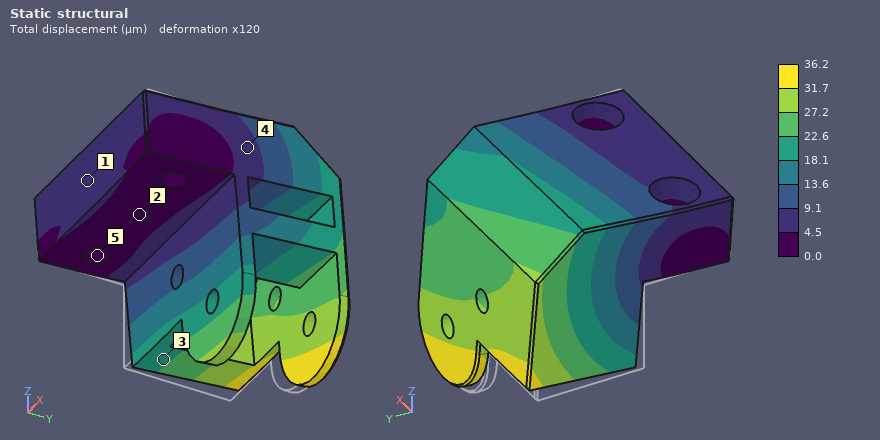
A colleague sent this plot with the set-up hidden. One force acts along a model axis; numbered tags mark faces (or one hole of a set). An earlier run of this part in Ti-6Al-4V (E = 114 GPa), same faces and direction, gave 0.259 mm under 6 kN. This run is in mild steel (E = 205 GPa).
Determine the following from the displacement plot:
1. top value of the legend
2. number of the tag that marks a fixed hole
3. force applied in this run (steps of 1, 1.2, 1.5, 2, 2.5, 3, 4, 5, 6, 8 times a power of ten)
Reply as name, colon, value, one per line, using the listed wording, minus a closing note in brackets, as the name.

top value of the legend: 36.2 µm
number of the tag that marks a fixed hole: 5
force applied in this run: 1.5 kN
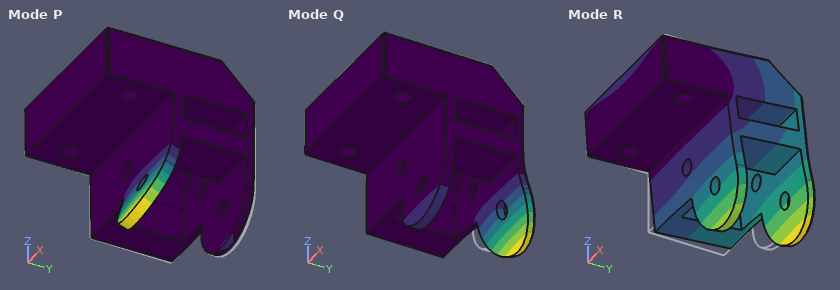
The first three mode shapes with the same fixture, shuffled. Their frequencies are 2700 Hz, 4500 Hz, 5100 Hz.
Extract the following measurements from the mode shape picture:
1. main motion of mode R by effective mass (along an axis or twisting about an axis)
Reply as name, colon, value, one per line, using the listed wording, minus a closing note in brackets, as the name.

main motion of mode R by effective mass: along Z
